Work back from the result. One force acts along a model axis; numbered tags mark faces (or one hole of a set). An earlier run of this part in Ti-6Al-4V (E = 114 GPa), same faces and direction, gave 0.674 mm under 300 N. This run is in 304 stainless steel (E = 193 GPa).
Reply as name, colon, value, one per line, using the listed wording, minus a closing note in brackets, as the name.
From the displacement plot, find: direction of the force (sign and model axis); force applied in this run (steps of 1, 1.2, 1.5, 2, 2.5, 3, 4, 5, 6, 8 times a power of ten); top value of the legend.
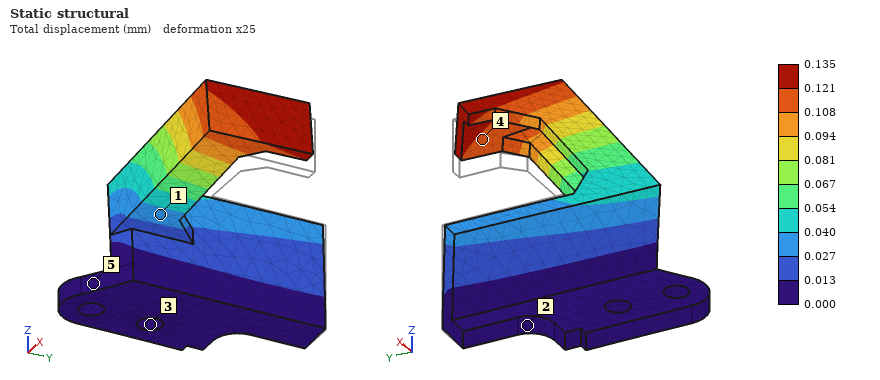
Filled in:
direction of the force: +Z
force applied in this run: 100 N
top value of the legend: 0.135 mm
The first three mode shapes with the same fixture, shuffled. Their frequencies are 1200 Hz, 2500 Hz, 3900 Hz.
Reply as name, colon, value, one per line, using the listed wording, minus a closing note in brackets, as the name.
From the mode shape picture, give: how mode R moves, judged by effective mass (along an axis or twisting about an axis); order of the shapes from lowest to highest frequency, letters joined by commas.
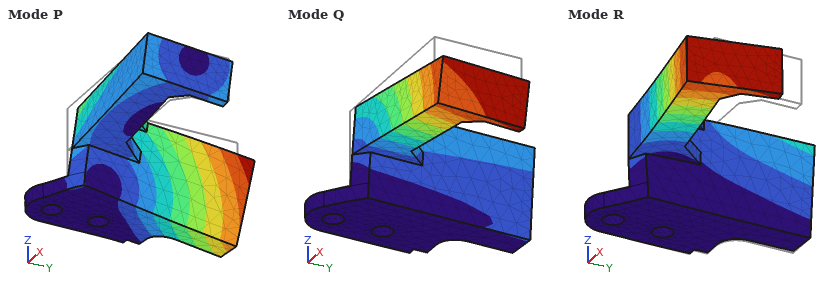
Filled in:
how mode R moves, judged by effective mass: along Y
order of the shapes from lowest to highest frequency, letters joined by commas: Q, R, P
